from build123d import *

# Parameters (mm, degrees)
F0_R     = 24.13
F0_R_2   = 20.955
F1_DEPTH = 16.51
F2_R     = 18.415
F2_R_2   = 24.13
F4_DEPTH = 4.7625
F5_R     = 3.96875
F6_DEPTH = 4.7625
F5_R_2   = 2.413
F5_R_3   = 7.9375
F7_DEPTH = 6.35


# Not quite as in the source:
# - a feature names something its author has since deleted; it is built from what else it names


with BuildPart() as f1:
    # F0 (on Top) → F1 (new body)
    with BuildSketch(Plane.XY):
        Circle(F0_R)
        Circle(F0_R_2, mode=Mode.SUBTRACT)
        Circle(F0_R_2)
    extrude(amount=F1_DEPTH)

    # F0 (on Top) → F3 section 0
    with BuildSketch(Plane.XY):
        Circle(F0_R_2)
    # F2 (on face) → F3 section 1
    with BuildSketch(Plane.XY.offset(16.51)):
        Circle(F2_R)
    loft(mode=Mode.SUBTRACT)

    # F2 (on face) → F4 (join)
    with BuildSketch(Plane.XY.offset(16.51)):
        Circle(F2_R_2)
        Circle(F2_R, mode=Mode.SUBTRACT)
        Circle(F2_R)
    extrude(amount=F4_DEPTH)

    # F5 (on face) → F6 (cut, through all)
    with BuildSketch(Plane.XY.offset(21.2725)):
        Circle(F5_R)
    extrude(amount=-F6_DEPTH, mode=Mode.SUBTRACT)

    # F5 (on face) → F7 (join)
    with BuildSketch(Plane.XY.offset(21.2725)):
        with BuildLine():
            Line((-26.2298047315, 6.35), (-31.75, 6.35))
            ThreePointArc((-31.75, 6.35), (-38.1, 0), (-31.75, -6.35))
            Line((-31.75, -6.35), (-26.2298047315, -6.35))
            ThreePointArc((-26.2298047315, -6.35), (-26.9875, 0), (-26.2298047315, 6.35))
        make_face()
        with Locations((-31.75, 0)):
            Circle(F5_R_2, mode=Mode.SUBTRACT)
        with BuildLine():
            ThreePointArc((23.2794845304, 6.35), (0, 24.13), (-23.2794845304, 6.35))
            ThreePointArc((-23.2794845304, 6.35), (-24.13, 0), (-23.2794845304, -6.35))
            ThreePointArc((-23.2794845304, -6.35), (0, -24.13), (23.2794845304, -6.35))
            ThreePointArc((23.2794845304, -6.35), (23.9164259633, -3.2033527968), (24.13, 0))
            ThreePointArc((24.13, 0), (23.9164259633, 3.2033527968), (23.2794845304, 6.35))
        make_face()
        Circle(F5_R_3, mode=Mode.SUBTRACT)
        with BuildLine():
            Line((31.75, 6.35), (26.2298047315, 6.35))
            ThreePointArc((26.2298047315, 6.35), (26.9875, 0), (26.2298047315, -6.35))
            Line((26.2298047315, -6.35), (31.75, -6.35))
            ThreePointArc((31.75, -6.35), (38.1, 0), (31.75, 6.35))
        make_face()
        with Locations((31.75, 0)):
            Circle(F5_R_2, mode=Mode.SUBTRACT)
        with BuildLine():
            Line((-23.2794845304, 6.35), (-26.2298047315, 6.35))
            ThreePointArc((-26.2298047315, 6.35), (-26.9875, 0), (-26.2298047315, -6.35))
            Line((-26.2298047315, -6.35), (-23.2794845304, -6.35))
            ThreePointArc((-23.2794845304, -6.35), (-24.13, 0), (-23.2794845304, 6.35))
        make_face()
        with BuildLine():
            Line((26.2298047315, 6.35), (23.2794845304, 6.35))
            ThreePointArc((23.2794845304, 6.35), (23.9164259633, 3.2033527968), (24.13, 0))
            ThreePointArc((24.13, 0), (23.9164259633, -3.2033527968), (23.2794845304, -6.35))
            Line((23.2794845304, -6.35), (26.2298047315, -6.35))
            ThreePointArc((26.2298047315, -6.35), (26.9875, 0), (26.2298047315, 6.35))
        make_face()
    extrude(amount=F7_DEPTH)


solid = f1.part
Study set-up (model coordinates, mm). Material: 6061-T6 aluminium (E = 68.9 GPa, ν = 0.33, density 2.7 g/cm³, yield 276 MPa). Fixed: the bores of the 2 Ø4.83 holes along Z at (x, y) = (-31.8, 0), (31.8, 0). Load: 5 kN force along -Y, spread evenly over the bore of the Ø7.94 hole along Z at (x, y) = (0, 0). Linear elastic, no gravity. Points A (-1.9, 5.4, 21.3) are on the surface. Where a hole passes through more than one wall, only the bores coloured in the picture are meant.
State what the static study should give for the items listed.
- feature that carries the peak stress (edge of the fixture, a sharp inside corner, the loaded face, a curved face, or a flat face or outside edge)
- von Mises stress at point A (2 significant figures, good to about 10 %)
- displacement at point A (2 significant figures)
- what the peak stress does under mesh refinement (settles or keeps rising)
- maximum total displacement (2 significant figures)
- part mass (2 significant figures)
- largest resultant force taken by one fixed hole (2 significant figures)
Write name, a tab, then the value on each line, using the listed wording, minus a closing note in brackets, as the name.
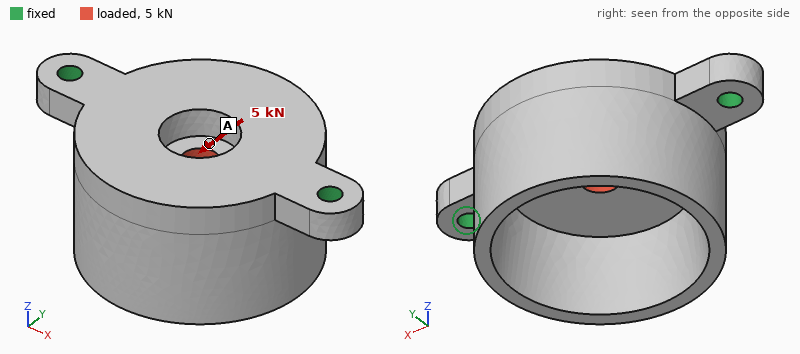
feature that carries the peak stress	edge of the fixture
von Mises stress at point A	42 MPa
displacement at point A	0.054 mm
what the peak stress does under mesh refinement	keeps rising
maximum total displacement	0.21 mm
part mass	83 g
largest resultant force taken by one fixed hole	2.5 kN
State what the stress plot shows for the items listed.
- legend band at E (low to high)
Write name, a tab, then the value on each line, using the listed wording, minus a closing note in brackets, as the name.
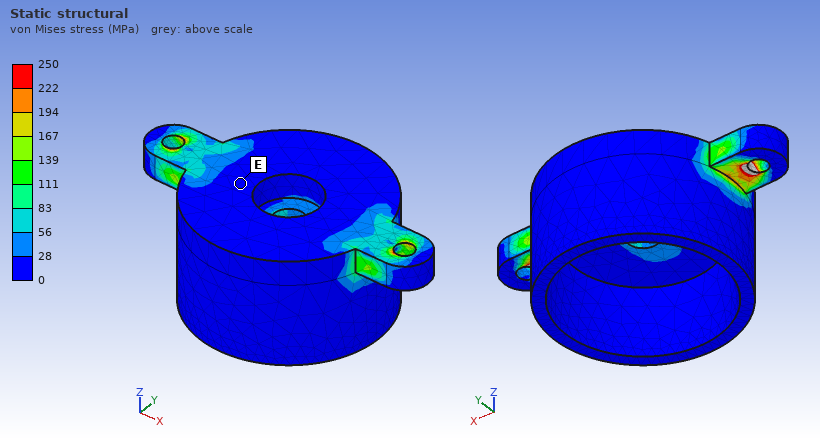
legend band at E	0 to 28 MPa
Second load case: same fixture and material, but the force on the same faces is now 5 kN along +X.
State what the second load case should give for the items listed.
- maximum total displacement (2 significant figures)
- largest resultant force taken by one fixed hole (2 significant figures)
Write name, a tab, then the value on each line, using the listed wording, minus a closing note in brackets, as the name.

maximum total displacement	12 µm
largest resultant force taken by one fixed hole	2.6 kN
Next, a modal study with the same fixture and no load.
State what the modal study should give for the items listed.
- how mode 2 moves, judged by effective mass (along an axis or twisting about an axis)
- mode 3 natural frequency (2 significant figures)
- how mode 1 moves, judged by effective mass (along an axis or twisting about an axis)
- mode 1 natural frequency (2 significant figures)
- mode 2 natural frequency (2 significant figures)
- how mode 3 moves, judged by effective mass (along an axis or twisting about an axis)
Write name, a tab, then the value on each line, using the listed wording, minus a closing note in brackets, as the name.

how mode 2 moves, judged by effective mass	along Z
mode 3 natural frequency	9900 Hz
how mode 1 moves, judged by effective mass	along Y
mode 1 natural frequency	2300 Hz
mode 2 natural frequency	6100 Hz
how mode 3 moves, judged by effective mass	along Y
